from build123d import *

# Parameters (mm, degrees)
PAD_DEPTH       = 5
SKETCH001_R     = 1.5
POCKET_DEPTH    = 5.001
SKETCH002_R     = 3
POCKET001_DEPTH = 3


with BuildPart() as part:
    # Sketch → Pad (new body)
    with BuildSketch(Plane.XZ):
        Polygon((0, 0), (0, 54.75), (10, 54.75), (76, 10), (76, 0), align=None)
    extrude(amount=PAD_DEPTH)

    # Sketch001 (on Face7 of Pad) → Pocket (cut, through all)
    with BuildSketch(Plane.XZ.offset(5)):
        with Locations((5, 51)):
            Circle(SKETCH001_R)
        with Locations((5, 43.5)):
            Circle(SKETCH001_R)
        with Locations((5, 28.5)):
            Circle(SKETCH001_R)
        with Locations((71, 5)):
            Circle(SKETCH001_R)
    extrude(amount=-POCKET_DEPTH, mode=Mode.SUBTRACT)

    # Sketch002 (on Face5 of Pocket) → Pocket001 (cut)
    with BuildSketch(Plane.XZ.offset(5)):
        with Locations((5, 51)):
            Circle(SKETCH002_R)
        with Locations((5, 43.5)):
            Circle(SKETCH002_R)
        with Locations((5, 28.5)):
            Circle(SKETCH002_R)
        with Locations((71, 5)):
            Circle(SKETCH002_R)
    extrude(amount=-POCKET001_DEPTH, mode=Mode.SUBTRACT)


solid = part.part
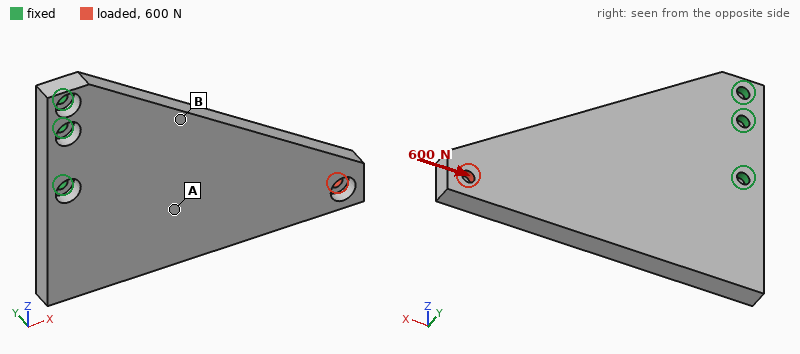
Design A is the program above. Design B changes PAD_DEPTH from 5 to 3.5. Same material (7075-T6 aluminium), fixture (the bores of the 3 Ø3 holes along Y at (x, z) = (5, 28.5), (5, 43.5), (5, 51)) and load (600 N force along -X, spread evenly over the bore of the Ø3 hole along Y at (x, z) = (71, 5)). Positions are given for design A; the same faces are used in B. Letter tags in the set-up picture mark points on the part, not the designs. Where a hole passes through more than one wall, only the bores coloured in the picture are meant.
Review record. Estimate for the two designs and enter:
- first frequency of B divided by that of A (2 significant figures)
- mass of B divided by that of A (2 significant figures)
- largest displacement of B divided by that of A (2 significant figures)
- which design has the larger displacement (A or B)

0.83
0.70
1.4
B
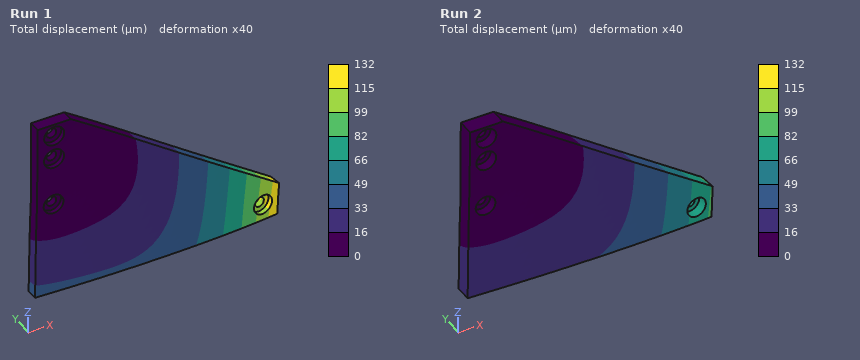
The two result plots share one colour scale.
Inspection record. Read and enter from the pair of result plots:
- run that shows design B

Run 1
